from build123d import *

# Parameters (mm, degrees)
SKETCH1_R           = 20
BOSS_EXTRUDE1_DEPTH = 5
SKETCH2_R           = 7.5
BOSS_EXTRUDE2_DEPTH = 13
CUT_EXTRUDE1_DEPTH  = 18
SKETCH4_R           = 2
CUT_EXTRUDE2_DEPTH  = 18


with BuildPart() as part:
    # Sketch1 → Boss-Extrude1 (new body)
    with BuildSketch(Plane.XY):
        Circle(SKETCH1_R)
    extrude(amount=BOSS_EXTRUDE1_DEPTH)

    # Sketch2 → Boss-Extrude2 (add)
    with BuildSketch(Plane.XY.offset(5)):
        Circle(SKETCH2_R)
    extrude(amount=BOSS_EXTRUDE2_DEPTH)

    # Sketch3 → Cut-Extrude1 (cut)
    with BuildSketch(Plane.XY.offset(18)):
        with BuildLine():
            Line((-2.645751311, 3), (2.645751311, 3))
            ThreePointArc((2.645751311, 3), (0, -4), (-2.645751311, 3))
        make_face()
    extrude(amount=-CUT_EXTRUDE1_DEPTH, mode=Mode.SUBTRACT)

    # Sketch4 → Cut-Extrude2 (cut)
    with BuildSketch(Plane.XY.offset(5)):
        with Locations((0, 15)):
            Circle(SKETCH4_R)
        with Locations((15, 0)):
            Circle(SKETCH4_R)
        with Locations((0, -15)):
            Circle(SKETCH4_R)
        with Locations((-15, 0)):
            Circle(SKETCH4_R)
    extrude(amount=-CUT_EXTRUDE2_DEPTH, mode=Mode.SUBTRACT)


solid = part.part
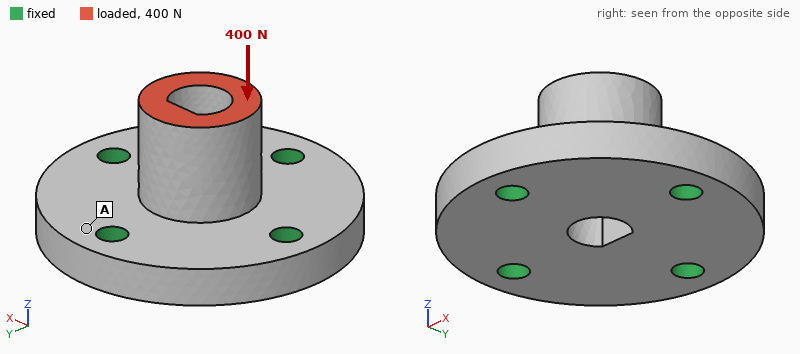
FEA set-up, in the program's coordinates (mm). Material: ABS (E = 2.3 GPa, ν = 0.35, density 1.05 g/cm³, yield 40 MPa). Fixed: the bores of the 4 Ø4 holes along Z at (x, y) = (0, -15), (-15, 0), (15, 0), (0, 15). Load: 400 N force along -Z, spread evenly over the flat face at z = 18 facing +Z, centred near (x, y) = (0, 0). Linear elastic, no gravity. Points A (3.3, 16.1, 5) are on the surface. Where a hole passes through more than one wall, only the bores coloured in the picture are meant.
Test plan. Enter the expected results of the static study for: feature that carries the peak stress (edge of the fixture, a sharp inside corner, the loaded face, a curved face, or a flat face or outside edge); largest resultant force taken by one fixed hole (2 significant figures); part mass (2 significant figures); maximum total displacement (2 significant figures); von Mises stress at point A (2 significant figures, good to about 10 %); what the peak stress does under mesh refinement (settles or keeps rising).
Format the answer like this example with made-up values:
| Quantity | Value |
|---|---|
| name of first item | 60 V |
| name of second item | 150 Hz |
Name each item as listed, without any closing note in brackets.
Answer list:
| Quantity | Value |
|---|---|
| feature that carries the peak stress | edge of the fixture |
| largest resultant force taken by one fixed hole | 110 N |
| part mass | 7.9 g |
| maximum total displacement | 57 µm |
| von Mises stress at point A | 1.9 MPa |
| what the peak stress does under mesh refinement | keeps rising |
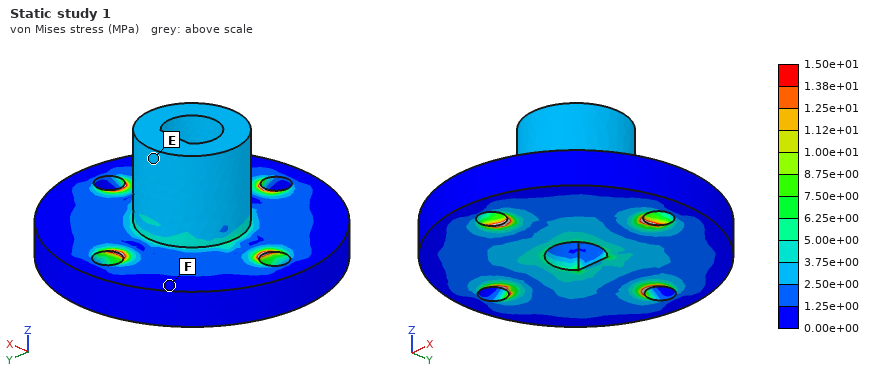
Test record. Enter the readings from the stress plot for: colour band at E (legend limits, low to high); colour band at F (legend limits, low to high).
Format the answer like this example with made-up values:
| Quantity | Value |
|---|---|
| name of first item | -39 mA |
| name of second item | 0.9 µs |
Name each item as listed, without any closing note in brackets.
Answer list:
| Quantity | Value |
|---|---|
| colour band at E | 2.50e+00 to 3.75e+00 MPa |
| colour band at F | 0.00e+00 to 1.25e+00 MPa |
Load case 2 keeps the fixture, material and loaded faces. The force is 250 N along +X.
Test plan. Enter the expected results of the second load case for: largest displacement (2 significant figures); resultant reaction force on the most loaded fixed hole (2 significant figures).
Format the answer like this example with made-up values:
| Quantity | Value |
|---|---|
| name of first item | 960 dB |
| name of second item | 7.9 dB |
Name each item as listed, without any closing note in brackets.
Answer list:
| Quantity | Value |
|---|---|
| largest displacement | 0.20 mm |
| resultant reaction force on the most loaded fixed hole | 170 N |
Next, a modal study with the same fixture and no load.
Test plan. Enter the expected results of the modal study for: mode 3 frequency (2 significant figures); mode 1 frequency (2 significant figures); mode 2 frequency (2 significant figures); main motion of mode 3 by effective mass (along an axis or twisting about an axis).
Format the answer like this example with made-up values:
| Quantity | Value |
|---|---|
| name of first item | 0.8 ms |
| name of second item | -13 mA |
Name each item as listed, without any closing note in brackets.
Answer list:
| Quantity | Value |
|---|---|
| mode 3 frequency | 8800 Hz |
| mode 1 frequency | 7000 Hz |
| mode 2 frequency | 7000 Hz |
| main motion of mode 3 by effective mass | along Z |
